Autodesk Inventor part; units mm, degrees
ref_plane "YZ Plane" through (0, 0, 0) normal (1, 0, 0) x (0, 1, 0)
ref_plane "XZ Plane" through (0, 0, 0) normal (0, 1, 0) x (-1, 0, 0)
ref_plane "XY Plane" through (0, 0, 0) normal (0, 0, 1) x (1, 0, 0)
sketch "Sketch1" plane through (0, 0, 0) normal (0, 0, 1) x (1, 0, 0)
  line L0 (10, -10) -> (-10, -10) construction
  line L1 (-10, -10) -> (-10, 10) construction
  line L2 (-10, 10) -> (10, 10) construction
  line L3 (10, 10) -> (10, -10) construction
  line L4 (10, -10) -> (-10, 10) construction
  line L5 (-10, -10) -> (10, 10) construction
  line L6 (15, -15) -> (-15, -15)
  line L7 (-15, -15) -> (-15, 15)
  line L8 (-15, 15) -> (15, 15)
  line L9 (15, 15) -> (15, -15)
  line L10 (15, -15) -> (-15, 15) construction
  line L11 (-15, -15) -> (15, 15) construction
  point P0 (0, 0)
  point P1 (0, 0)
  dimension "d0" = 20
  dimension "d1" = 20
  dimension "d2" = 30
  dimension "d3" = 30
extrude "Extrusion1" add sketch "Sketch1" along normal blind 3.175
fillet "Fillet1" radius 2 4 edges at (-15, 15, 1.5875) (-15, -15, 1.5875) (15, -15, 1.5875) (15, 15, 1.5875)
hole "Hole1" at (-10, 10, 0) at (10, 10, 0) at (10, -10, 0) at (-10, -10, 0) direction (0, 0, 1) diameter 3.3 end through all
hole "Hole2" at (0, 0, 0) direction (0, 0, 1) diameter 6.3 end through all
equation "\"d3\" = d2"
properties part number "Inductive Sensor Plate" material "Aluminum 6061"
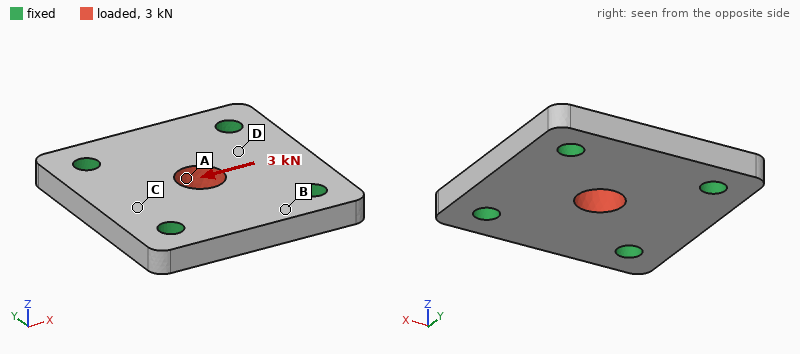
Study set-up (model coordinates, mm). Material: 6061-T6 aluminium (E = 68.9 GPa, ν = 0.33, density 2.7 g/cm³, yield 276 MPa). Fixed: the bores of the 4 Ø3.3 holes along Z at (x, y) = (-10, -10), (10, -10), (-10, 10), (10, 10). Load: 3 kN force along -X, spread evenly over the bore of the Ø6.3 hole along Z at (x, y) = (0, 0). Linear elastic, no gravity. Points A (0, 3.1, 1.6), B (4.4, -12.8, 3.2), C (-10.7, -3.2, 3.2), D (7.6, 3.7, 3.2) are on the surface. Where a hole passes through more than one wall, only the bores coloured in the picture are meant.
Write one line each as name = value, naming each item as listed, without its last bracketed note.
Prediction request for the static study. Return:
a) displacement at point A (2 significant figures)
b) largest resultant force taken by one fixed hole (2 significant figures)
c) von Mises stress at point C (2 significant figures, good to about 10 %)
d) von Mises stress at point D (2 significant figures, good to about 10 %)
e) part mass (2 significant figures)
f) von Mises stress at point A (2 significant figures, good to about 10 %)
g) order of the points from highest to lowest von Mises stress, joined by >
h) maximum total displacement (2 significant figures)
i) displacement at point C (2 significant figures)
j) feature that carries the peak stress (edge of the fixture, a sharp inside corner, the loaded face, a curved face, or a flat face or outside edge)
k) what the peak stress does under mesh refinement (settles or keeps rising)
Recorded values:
displacement at point A = 6.9 µm
largest resultant force taken by one fixed hole = 820 N
von Mises stress at point C = 18 MPa
von Mises stress at point D = 30 MPa
part mass = 7.1 g
von Mises stress at point A = 84 MPa
order of the points from highest to lowest von Mises stress, joined by > = A > D > C > B
maximum total displacement = 7.7 µm
displacement at point C = 4.1 µm
feature that carries the peak stress = edge of the fixture
what the peak stress does under mesh refinement = keeps rising
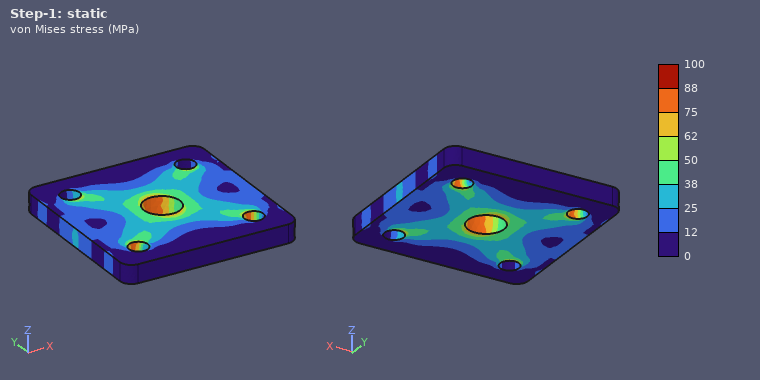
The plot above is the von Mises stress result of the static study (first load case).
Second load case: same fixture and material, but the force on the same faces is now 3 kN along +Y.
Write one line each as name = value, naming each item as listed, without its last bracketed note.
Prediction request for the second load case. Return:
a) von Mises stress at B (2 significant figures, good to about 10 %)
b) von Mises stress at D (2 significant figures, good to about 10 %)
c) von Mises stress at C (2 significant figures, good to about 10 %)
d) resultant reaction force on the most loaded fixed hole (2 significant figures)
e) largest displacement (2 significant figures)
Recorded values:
von Mises stress at B = 16 MPa
von Mises stress at D = 27 MPa
von Mises stress at C = 11 MPa
resultant reaction force on the most loaded fixed hole = 820 N
largest displacement = 7.7 µm
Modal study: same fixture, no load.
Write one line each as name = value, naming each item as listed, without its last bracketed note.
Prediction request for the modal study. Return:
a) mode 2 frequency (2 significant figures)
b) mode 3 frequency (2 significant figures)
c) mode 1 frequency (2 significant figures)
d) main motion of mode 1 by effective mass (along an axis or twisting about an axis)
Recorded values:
mode 2 frequency = 41 kHz
mode 3 frequency = 41 kHz
mode 1 frequency = 31 kHz
main motion of mode 1 by effective mass = along Z
